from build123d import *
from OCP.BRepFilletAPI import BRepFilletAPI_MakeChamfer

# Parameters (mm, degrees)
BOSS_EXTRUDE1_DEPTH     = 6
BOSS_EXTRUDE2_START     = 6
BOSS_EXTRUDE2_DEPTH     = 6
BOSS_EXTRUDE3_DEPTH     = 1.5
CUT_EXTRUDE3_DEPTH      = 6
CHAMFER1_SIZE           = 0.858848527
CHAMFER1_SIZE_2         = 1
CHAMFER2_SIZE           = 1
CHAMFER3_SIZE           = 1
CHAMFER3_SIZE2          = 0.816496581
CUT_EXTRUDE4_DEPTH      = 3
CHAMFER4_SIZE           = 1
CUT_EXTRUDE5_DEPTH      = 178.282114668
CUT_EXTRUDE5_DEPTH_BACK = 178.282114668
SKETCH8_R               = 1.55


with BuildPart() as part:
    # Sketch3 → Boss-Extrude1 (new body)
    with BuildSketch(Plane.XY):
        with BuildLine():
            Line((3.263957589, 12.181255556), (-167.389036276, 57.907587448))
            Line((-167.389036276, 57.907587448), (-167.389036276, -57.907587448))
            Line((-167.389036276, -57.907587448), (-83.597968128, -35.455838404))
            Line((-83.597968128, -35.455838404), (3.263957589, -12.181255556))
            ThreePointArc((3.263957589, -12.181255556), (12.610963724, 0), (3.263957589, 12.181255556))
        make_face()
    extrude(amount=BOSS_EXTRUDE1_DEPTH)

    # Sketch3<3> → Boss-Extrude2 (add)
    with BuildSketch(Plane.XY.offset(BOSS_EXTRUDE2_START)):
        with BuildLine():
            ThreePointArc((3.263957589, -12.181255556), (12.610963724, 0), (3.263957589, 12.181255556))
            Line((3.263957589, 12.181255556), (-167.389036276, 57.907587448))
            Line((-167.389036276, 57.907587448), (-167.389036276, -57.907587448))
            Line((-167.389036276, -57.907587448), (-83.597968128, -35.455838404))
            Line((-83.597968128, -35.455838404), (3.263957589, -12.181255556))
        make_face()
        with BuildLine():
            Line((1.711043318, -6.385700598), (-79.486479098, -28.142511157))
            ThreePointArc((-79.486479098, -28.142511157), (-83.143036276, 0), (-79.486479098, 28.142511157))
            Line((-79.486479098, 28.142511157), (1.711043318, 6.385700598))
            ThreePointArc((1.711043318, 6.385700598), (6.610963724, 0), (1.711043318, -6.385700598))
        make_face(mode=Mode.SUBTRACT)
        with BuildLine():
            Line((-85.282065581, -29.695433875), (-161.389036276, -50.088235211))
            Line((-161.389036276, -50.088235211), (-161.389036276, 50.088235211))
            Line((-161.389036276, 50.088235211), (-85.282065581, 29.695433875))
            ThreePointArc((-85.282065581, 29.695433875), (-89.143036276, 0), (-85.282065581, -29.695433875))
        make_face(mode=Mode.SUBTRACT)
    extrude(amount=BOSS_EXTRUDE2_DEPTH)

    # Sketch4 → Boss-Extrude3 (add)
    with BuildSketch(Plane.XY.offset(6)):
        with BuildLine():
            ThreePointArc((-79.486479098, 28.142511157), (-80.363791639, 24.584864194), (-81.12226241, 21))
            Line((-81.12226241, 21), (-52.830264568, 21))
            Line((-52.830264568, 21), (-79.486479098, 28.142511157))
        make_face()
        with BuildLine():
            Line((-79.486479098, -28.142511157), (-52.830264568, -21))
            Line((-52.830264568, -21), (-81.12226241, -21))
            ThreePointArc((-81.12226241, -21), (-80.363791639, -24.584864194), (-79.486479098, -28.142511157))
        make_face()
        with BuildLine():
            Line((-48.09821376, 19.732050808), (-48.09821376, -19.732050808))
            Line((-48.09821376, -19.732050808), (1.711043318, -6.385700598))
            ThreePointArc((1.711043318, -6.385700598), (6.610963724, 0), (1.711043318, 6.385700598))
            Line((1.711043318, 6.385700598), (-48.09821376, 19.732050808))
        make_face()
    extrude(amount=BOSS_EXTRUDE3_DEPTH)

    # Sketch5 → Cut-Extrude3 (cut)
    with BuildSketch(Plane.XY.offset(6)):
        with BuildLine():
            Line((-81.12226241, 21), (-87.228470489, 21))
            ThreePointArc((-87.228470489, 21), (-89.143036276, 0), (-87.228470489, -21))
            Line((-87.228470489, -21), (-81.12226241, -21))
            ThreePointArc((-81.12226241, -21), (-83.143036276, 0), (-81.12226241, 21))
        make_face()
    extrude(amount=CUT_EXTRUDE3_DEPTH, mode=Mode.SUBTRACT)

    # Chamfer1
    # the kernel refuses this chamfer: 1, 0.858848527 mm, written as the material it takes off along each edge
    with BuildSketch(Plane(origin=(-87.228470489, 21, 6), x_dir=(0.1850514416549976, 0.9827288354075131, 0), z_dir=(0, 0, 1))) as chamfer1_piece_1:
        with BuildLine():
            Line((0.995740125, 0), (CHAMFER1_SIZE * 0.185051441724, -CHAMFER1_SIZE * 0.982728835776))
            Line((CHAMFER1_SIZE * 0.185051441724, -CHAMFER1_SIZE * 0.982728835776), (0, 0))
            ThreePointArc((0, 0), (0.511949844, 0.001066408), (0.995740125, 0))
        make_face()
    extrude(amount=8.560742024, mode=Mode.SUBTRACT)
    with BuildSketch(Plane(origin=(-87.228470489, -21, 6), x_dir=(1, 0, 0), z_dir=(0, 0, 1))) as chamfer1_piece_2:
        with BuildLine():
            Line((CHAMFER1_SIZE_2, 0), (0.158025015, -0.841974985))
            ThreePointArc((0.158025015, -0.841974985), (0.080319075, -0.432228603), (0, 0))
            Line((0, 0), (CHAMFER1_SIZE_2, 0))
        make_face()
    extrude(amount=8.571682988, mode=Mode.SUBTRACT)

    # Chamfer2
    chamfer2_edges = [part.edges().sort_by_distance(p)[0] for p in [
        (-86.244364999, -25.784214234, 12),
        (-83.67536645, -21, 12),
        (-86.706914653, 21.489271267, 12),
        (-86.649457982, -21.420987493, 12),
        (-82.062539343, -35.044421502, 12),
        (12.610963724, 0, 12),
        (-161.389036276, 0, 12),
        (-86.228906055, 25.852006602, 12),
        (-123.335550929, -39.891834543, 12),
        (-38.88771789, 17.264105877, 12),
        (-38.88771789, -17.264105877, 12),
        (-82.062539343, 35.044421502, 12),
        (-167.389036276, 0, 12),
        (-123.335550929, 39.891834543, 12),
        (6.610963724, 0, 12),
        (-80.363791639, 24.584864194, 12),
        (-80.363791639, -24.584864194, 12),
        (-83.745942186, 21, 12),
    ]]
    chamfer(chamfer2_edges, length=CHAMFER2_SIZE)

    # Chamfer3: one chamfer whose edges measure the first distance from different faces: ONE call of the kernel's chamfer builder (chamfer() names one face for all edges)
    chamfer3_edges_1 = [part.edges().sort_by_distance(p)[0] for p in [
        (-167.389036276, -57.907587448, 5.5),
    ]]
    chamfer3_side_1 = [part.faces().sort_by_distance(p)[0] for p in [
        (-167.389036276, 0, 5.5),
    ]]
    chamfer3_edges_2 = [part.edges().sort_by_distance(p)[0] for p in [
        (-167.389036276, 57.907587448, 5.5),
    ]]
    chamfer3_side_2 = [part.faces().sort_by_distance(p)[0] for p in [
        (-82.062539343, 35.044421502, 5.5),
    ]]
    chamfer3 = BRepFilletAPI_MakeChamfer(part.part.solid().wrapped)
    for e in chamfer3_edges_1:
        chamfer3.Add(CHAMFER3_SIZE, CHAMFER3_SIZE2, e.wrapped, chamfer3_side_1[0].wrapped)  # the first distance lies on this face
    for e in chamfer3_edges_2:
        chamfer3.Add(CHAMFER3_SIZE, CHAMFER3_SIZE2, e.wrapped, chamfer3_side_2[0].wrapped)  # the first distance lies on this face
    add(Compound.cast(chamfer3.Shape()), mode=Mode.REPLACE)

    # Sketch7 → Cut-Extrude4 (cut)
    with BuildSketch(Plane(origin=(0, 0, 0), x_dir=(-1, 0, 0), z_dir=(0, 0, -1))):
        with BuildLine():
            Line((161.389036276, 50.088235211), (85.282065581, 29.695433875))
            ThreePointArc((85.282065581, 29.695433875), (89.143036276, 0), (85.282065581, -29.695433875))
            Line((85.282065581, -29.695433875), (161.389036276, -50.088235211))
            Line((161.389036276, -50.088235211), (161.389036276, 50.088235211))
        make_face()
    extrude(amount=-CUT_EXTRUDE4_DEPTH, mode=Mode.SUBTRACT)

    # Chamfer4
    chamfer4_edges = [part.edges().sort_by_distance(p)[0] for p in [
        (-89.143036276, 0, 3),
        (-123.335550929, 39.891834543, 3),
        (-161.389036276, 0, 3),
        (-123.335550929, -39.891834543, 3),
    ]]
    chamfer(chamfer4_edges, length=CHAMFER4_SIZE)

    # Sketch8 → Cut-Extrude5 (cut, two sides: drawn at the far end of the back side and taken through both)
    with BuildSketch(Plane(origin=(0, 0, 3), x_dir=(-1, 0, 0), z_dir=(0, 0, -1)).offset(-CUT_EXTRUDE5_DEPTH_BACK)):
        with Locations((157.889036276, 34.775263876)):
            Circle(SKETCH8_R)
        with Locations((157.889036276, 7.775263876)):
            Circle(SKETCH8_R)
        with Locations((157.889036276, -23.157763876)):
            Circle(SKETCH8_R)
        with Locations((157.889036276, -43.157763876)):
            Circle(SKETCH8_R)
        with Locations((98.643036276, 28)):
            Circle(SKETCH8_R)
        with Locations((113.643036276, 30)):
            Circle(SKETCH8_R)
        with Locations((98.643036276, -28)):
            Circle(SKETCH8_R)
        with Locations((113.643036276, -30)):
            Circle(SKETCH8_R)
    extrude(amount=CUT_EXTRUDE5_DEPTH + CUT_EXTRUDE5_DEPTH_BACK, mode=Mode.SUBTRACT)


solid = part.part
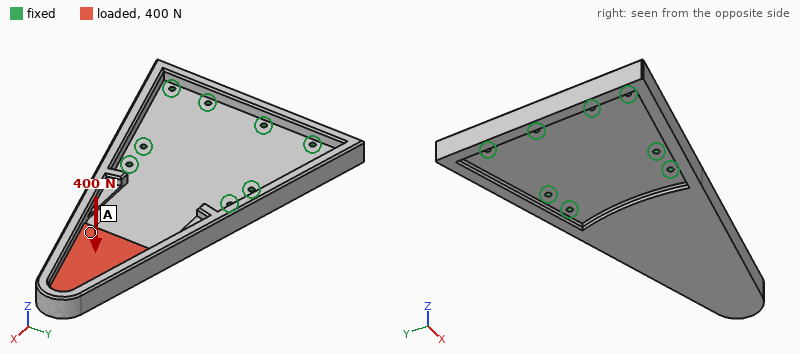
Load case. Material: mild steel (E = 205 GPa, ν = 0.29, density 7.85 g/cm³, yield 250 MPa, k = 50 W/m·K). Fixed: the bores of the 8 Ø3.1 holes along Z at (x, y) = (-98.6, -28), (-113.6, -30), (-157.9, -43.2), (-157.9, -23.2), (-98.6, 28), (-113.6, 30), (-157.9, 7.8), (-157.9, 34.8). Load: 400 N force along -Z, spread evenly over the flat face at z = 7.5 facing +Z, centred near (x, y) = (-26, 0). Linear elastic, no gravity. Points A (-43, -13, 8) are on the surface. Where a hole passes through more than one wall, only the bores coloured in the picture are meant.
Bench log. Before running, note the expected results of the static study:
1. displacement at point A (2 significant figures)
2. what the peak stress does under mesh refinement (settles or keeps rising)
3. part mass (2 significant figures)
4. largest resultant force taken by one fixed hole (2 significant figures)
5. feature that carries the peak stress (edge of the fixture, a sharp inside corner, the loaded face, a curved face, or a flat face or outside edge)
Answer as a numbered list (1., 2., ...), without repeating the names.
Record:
1. 0.12 mm
2. keeps rising
3. 590 g
4. 770 N
5. edge of the fixture
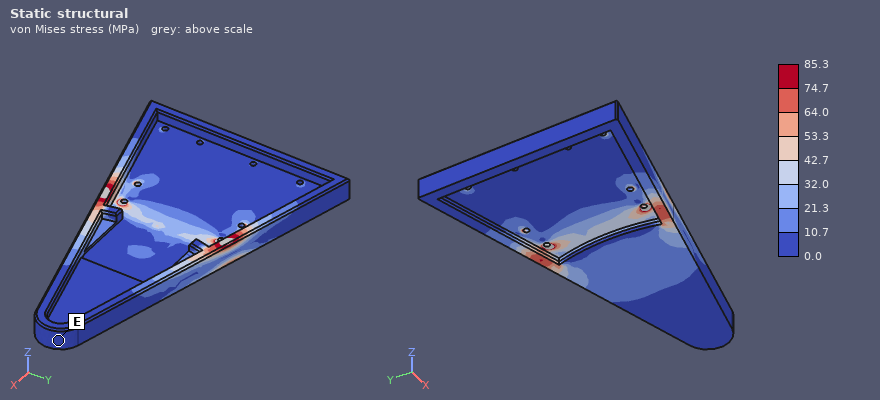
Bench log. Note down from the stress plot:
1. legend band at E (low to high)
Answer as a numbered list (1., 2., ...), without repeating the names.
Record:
1. 0.0 to 10.7 MPa
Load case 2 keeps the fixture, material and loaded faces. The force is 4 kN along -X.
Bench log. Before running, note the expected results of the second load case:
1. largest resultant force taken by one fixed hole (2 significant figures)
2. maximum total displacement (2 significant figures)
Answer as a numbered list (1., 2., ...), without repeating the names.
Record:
1. 1.1 kN
2. 0.16 mm
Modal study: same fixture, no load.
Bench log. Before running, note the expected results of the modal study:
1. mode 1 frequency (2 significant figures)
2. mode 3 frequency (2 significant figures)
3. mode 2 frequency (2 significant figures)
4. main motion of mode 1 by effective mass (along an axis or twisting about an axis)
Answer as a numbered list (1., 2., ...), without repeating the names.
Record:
1. 530 Hz
2. 3300 Hz
3. 2700 Hz
4. along Z
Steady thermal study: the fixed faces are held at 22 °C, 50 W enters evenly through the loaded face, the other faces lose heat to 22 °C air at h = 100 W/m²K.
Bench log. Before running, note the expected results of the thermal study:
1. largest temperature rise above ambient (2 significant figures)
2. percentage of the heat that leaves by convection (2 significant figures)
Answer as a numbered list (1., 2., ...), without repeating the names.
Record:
1. 64 K
2. 87 %
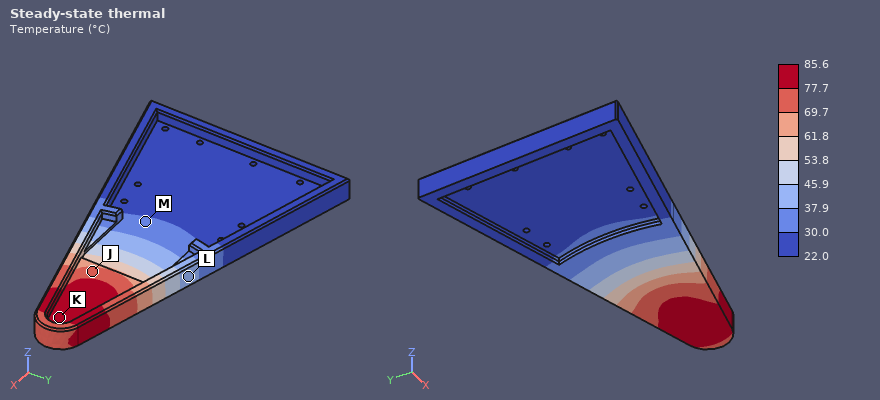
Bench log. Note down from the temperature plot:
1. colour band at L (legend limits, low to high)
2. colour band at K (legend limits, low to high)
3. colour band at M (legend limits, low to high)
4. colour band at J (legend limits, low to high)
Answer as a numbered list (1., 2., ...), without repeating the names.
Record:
1. 37.9 to 45.9 °C
2. 77.7 to 85.6 °C
3. 30.0 to 37.9 °C
4. 69.7 to 77.7 °C
